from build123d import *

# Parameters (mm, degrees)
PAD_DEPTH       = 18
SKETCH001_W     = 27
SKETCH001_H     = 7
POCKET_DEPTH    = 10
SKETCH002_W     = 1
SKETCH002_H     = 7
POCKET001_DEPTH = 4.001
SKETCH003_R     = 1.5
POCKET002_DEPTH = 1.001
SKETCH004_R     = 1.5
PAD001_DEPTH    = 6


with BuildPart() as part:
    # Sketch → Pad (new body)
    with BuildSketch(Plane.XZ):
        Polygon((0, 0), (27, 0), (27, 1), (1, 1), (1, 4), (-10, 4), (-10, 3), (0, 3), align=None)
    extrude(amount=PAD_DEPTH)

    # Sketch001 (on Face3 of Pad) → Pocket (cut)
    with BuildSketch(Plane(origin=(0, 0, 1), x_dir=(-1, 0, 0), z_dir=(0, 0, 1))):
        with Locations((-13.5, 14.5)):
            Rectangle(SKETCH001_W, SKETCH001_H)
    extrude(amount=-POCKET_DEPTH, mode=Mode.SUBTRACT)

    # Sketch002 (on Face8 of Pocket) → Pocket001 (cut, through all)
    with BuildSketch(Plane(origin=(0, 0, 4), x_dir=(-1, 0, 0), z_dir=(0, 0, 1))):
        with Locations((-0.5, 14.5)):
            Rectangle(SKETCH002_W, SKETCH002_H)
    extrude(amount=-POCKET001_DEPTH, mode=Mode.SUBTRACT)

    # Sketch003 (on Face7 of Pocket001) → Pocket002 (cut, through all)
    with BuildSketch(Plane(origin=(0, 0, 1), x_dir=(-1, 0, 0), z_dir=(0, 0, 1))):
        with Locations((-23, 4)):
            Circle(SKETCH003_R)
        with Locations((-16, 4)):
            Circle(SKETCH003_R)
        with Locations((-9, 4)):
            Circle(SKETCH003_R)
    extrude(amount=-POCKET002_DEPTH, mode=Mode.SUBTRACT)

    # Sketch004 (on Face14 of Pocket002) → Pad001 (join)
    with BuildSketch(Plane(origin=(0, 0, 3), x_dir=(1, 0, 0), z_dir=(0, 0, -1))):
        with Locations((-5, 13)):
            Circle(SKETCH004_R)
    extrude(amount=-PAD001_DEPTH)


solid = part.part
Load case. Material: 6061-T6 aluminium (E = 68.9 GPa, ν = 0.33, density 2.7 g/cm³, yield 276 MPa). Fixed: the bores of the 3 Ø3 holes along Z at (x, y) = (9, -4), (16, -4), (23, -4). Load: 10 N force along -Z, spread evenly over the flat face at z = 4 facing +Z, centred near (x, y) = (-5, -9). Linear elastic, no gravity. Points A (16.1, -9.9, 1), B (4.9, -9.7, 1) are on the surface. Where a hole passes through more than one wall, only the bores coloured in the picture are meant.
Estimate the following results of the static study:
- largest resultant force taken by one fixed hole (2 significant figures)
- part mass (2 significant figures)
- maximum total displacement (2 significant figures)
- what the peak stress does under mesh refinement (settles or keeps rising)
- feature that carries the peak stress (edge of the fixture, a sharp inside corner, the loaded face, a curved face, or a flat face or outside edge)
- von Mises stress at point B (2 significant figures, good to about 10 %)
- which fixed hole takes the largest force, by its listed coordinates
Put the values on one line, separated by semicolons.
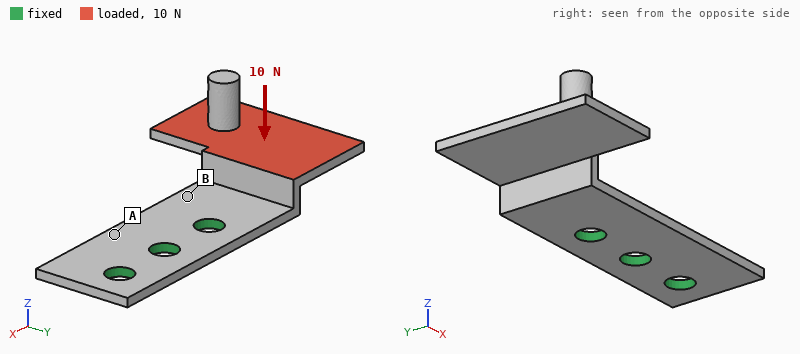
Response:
13 N; 1.4 g; 0.26 mm; keeps rising; edge of the fixture; 47 MPa; (9, -4)
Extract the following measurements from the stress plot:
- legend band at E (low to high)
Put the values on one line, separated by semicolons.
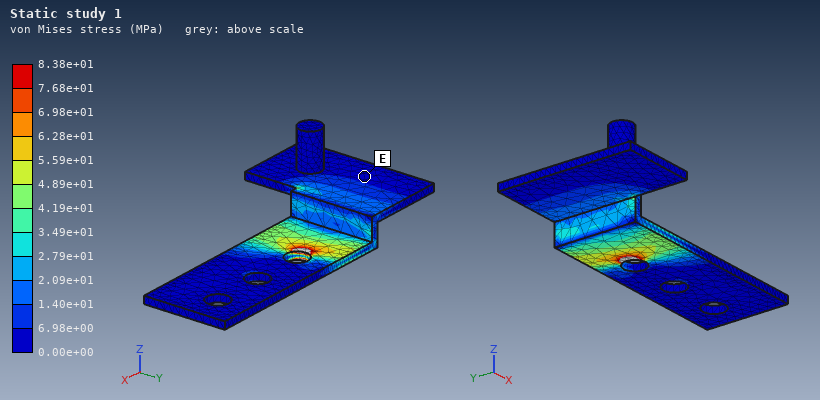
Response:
0.00e+00 to 6.98e+00 MPa
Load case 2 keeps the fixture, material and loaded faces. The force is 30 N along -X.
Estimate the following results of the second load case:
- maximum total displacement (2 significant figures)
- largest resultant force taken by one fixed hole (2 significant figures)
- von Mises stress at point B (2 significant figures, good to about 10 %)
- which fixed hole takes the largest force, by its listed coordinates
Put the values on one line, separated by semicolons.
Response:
0.24 mm; 21 N; 60 MPa; (9, -4)
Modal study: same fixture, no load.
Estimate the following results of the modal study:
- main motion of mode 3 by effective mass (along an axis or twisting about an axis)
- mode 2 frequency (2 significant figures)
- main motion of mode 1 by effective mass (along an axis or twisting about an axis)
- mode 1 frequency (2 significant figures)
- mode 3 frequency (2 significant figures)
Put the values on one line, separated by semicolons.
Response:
along Y; 3700 Hz; along Z; 1500 Hz; 6000 Hz
